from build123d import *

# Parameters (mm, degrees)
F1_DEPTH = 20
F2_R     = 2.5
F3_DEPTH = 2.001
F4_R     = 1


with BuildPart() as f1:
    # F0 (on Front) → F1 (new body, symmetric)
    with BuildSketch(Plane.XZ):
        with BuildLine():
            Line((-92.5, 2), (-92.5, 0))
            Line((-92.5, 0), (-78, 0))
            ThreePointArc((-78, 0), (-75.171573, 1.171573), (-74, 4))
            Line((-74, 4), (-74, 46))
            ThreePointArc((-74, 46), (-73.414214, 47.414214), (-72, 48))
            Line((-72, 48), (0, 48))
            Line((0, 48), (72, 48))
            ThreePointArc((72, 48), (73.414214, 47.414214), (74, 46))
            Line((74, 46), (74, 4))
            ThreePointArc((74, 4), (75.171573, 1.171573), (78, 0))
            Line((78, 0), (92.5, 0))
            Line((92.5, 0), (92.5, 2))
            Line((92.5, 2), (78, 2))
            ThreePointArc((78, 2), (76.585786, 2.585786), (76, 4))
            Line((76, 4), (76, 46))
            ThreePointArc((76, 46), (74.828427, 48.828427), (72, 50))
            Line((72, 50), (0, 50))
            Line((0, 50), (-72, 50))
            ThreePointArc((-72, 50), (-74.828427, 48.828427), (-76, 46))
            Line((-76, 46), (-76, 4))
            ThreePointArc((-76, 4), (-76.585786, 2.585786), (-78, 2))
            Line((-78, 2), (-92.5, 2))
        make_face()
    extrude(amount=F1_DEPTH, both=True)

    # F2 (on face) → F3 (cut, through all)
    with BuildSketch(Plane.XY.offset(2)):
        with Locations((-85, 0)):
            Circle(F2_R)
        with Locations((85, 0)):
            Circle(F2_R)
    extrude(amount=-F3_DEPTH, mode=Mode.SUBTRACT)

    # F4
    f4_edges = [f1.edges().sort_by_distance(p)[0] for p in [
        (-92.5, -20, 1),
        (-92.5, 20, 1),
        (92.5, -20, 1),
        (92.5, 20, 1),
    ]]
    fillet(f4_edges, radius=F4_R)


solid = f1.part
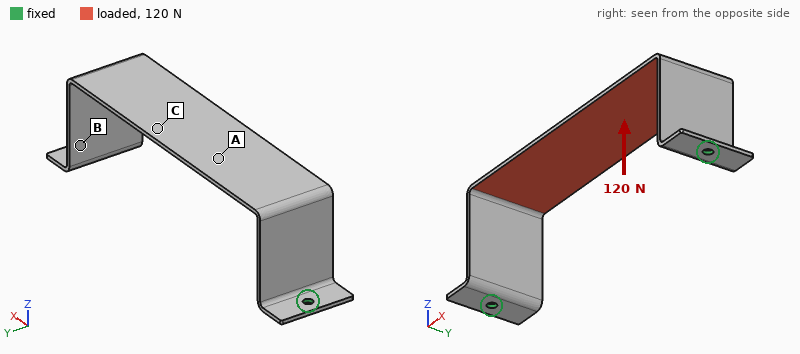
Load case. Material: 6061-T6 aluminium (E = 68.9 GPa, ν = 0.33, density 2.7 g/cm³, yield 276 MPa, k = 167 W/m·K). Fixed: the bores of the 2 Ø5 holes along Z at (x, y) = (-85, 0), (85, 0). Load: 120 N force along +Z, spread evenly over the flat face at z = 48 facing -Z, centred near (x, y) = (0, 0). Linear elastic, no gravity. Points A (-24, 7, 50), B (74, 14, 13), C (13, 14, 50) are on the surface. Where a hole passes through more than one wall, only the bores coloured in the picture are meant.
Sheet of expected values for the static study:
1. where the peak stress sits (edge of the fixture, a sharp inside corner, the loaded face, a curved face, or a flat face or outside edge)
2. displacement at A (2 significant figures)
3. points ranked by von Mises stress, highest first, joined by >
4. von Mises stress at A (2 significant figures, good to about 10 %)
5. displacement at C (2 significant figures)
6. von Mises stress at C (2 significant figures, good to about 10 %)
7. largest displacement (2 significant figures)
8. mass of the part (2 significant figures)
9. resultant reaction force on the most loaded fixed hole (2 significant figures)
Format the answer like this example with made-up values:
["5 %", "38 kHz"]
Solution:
["a curved face", "0.72 mm", "C > A > B", "27 MPa", "0.83 mm", "33 MPa", "0.89 mm", "59 g", "72 N"]
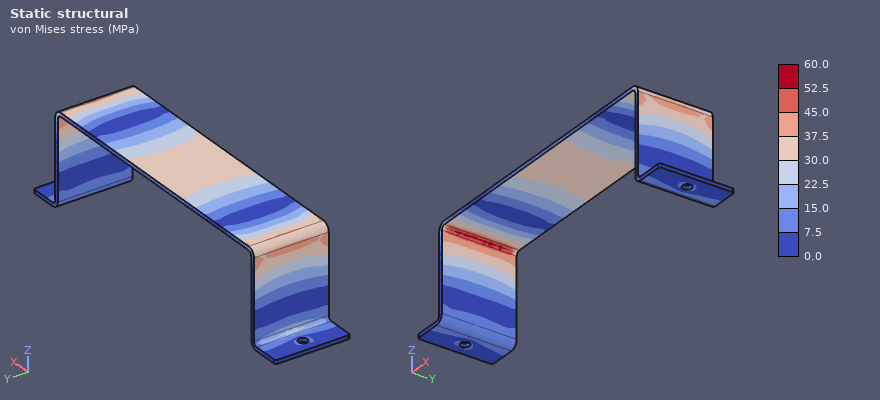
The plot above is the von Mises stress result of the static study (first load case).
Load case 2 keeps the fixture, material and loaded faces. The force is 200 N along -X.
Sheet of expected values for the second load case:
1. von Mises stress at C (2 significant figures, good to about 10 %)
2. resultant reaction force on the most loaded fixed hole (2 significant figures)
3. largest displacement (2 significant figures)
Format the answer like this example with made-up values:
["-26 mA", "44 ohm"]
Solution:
["14 MPa", "100 N", "1.4 mm"]
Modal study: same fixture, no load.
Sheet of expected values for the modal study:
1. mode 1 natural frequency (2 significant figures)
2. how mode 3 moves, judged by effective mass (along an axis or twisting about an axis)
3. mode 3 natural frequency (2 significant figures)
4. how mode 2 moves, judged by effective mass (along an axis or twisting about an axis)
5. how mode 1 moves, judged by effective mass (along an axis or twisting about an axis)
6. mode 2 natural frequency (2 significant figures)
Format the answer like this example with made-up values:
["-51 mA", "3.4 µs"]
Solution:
["300 Hz", "along Y", "410 Hz", "along Z", "along X", "380 Hz"]
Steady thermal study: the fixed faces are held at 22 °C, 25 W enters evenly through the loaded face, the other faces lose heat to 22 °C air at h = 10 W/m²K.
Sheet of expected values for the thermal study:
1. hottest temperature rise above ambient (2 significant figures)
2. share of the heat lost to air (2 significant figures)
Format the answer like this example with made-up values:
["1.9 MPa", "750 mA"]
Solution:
["74 K", "26 %"]
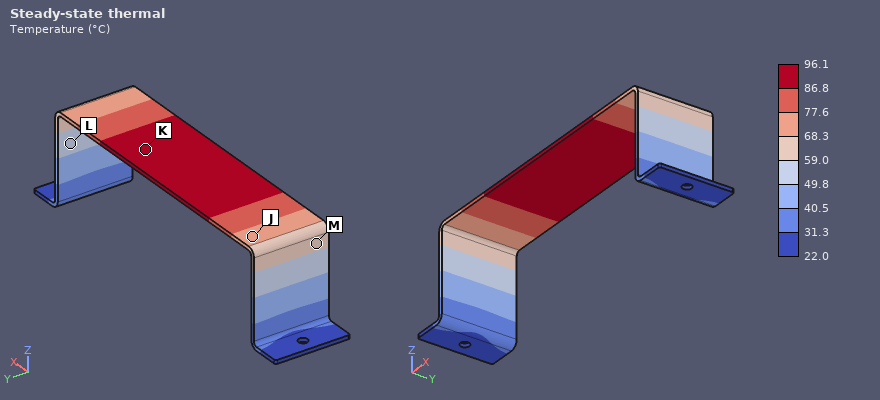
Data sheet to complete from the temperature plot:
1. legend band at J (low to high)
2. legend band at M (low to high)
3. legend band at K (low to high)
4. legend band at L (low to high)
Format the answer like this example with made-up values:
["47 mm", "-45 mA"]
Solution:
["68.3 to 77.6 °C", "59.0 to 68.3 °C", "86.8 to 96.1 °C", "49.8 to 59.0 °C"]
